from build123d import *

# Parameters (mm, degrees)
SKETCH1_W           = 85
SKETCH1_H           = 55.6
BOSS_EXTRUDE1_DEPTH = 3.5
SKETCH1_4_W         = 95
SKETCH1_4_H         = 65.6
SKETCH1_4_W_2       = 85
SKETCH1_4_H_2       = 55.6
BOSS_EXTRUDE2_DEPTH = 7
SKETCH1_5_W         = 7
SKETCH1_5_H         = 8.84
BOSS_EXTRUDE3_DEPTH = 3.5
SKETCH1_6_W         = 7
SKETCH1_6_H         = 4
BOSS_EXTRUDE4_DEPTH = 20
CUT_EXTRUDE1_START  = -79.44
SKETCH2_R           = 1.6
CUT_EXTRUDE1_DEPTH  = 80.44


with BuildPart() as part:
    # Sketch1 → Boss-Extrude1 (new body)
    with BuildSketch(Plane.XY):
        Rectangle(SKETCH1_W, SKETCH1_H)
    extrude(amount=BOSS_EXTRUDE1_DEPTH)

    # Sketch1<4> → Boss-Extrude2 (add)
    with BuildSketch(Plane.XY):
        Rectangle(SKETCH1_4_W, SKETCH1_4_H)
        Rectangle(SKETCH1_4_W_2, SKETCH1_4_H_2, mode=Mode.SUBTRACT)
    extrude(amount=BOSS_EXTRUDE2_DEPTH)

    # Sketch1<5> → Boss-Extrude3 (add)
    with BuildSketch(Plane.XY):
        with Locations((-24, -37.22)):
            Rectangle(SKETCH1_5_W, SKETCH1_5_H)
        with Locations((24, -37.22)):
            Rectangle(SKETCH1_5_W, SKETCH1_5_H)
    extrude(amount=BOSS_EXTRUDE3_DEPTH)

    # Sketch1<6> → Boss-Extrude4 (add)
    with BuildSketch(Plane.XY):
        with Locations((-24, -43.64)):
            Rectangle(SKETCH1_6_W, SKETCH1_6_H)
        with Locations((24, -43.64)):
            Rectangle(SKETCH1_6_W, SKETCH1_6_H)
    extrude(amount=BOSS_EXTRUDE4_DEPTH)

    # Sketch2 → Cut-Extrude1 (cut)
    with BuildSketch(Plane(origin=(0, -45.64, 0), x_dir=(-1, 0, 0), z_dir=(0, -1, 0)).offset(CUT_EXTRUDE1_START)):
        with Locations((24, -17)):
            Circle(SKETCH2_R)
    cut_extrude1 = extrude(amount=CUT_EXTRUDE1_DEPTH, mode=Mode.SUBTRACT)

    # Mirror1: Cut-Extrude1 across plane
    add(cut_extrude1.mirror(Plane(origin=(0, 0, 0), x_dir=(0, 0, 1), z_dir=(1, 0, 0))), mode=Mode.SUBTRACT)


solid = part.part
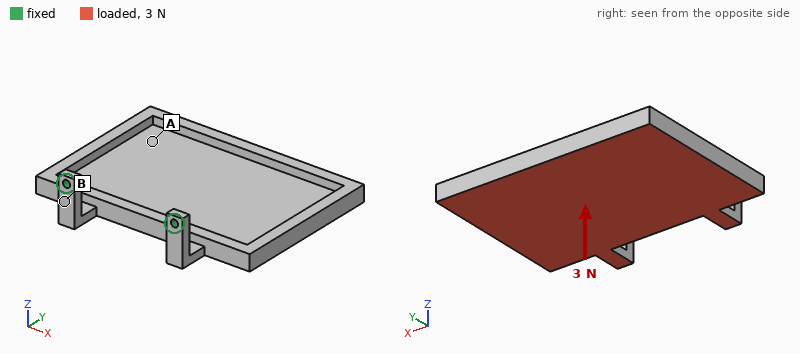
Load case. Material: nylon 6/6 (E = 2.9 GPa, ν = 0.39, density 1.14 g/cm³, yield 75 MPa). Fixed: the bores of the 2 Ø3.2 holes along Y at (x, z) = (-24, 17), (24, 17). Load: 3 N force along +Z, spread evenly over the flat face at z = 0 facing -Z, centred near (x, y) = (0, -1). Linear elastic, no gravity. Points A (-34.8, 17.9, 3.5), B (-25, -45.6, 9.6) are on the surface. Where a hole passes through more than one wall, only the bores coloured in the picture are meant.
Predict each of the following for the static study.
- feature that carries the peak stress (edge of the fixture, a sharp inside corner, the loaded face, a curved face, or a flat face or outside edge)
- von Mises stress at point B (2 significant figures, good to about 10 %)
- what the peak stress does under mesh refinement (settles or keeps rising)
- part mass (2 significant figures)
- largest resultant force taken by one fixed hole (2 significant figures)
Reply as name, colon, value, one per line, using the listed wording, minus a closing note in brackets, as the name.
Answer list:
feature that carries the peak stress: edge of the fixture
von Mises stress at point B: 3.4 MPa
what the peak stress does under mesh refinement: keeps rising
part mass: 33 g
largest resultant force taken by one fixed hole: 1.5 N
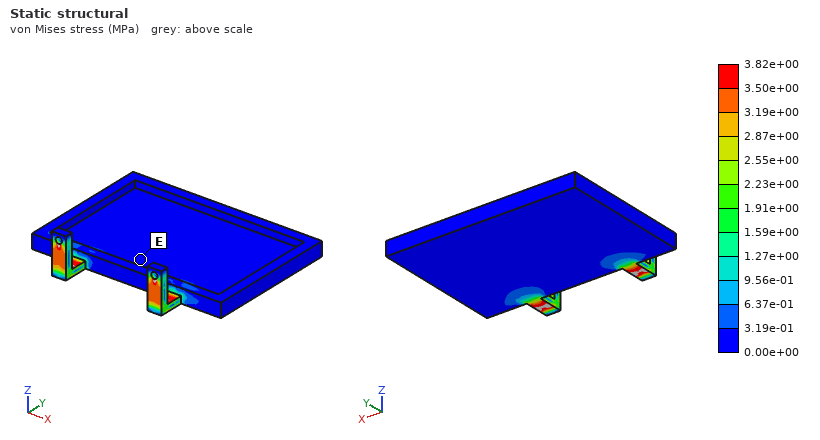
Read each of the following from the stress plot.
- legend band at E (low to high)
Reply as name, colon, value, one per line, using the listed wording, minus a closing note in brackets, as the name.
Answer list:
legend band at E: 0.00e+00 to 3.19e-01 MPa
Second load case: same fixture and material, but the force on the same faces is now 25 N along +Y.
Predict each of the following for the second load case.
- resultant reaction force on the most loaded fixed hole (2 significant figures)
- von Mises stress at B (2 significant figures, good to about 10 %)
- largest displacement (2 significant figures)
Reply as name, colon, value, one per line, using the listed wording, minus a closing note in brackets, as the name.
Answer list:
resultant reaction force on the most loaded fixed hole: 13 N
von Mises stress at B: 6.4 MPa
largest displacement: 1.4 mm
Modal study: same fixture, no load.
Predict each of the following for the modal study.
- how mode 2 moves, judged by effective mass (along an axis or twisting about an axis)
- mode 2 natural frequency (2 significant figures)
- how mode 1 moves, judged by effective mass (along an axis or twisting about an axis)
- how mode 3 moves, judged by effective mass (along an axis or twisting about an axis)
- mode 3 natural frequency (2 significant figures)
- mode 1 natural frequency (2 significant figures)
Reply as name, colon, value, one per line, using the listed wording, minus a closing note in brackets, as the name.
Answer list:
how mode 2 moves, judged by effective mass: along X
mode 2 natural frequency: 180 Hz
how mode 1 moves, judged by effective mass: along Z
how mode 3 moves, judged by effective mass: along X
mode 3 natural frequency: 260 Hz
mode 1 natural frequency: 52 Hz
